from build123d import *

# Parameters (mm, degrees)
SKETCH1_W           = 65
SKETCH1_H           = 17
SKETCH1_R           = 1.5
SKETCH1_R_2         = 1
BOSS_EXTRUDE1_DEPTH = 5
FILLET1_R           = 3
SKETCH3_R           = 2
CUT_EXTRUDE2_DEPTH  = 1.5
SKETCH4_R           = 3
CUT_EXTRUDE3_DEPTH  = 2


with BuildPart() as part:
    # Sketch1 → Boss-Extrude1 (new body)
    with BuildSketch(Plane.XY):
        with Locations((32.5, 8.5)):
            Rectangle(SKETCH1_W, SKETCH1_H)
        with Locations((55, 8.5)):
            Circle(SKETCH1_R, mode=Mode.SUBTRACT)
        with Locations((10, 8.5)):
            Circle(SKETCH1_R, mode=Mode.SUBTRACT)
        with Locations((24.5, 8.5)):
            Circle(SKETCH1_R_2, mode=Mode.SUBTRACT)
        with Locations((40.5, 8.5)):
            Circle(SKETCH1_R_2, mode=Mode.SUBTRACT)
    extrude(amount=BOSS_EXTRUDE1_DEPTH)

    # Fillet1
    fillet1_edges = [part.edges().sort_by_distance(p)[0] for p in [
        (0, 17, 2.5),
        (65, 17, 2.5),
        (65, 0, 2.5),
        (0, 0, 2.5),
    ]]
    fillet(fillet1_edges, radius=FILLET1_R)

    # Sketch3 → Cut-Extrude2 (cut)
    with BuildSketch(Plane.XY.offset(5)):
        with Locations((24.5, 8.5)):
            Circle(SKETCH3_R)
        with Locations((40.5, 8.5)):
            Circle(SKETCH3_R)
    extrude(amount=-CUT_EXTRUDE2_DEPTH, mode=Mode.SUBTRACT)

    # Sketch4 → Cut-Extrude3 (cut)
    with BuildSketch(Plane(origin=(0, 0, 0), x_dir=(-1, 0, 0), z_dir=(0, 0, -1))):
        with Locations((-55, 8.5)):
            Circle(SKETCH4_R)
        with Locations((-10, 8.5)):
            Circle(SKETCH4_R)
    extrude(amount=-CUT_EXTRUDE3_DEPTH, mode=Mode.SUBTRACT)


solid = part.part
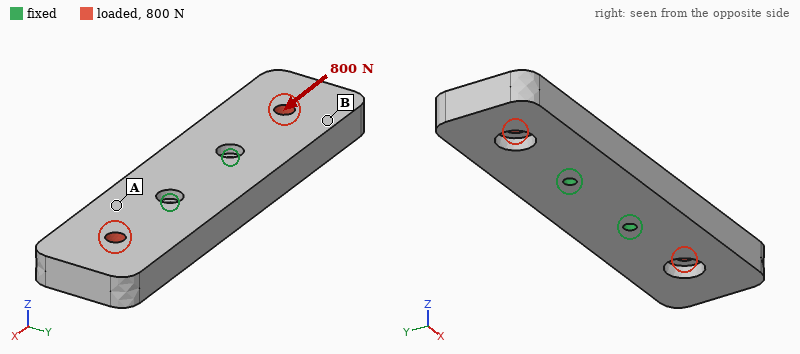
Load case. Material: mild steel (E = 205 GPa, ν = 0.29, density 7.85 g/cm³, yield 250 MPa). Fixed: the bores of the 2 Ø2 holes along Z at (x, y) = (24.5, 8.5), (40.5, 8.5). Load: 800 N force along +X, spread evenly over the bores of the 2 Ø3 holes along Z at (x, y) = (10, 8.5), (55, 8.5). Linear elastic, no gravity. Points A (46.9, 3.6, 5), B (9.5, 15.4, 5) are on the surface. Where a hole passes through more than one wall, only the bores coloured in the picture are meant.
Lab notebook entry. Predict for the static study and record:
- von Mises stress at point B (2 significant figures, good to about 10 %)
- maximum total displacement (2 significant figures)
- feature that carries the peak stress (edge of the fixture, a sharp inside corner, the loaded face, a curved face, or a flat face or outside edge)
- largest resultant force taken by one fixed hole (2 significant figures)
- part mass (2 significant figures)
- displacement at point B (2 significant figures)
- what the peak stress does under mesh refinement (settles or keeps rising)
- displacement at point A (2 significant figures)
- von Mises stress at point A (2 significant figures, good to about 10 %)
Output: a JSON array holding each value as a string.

["4.8 MPa", "4.3 µm", "edge of the fixture", "400 N", "41 g", "2.3 µm", "keeps rising", "0.95 µm", "10 MPa"]
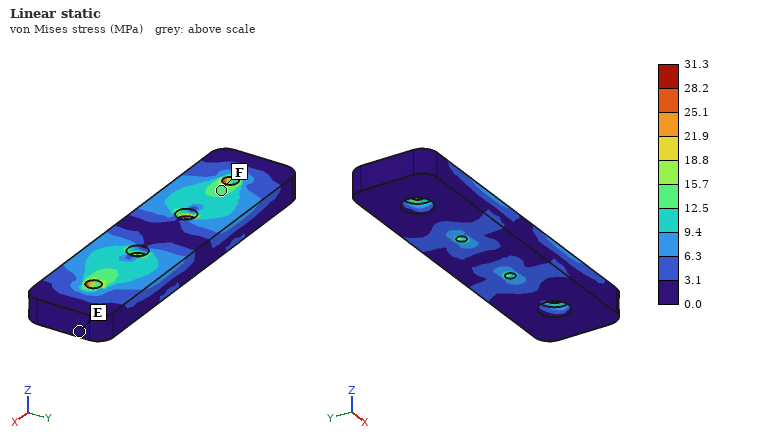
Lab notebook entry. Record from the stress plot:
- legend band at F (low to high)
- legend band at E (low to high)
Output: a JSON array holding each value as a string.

["12.5 to 15.7 MPa", "0.0 to 3.1 MPa"]
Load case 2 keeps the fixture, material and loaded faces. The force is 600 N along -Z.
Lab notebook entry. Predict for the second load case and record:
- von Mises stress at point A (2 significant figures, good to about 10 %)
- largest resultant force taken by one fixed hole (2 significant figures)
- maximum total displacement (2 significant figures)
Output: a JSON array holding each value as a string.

["35 MPa", "460 N", "29 µm"]
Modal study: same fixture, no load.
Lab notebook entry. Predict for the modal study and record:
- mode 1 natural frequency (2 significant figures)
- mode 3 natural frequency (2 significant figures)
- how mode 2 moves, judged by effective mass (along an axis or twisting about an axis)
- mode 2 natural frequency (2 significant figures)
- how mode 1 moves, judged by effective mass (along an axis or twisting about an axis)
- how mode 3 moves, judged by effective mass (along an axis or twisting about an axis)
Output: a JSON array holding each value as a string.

["5500 Hz", "11 kHz", "twisting about Y", "5700 Hz", "along Z", "twisting about Z"]
